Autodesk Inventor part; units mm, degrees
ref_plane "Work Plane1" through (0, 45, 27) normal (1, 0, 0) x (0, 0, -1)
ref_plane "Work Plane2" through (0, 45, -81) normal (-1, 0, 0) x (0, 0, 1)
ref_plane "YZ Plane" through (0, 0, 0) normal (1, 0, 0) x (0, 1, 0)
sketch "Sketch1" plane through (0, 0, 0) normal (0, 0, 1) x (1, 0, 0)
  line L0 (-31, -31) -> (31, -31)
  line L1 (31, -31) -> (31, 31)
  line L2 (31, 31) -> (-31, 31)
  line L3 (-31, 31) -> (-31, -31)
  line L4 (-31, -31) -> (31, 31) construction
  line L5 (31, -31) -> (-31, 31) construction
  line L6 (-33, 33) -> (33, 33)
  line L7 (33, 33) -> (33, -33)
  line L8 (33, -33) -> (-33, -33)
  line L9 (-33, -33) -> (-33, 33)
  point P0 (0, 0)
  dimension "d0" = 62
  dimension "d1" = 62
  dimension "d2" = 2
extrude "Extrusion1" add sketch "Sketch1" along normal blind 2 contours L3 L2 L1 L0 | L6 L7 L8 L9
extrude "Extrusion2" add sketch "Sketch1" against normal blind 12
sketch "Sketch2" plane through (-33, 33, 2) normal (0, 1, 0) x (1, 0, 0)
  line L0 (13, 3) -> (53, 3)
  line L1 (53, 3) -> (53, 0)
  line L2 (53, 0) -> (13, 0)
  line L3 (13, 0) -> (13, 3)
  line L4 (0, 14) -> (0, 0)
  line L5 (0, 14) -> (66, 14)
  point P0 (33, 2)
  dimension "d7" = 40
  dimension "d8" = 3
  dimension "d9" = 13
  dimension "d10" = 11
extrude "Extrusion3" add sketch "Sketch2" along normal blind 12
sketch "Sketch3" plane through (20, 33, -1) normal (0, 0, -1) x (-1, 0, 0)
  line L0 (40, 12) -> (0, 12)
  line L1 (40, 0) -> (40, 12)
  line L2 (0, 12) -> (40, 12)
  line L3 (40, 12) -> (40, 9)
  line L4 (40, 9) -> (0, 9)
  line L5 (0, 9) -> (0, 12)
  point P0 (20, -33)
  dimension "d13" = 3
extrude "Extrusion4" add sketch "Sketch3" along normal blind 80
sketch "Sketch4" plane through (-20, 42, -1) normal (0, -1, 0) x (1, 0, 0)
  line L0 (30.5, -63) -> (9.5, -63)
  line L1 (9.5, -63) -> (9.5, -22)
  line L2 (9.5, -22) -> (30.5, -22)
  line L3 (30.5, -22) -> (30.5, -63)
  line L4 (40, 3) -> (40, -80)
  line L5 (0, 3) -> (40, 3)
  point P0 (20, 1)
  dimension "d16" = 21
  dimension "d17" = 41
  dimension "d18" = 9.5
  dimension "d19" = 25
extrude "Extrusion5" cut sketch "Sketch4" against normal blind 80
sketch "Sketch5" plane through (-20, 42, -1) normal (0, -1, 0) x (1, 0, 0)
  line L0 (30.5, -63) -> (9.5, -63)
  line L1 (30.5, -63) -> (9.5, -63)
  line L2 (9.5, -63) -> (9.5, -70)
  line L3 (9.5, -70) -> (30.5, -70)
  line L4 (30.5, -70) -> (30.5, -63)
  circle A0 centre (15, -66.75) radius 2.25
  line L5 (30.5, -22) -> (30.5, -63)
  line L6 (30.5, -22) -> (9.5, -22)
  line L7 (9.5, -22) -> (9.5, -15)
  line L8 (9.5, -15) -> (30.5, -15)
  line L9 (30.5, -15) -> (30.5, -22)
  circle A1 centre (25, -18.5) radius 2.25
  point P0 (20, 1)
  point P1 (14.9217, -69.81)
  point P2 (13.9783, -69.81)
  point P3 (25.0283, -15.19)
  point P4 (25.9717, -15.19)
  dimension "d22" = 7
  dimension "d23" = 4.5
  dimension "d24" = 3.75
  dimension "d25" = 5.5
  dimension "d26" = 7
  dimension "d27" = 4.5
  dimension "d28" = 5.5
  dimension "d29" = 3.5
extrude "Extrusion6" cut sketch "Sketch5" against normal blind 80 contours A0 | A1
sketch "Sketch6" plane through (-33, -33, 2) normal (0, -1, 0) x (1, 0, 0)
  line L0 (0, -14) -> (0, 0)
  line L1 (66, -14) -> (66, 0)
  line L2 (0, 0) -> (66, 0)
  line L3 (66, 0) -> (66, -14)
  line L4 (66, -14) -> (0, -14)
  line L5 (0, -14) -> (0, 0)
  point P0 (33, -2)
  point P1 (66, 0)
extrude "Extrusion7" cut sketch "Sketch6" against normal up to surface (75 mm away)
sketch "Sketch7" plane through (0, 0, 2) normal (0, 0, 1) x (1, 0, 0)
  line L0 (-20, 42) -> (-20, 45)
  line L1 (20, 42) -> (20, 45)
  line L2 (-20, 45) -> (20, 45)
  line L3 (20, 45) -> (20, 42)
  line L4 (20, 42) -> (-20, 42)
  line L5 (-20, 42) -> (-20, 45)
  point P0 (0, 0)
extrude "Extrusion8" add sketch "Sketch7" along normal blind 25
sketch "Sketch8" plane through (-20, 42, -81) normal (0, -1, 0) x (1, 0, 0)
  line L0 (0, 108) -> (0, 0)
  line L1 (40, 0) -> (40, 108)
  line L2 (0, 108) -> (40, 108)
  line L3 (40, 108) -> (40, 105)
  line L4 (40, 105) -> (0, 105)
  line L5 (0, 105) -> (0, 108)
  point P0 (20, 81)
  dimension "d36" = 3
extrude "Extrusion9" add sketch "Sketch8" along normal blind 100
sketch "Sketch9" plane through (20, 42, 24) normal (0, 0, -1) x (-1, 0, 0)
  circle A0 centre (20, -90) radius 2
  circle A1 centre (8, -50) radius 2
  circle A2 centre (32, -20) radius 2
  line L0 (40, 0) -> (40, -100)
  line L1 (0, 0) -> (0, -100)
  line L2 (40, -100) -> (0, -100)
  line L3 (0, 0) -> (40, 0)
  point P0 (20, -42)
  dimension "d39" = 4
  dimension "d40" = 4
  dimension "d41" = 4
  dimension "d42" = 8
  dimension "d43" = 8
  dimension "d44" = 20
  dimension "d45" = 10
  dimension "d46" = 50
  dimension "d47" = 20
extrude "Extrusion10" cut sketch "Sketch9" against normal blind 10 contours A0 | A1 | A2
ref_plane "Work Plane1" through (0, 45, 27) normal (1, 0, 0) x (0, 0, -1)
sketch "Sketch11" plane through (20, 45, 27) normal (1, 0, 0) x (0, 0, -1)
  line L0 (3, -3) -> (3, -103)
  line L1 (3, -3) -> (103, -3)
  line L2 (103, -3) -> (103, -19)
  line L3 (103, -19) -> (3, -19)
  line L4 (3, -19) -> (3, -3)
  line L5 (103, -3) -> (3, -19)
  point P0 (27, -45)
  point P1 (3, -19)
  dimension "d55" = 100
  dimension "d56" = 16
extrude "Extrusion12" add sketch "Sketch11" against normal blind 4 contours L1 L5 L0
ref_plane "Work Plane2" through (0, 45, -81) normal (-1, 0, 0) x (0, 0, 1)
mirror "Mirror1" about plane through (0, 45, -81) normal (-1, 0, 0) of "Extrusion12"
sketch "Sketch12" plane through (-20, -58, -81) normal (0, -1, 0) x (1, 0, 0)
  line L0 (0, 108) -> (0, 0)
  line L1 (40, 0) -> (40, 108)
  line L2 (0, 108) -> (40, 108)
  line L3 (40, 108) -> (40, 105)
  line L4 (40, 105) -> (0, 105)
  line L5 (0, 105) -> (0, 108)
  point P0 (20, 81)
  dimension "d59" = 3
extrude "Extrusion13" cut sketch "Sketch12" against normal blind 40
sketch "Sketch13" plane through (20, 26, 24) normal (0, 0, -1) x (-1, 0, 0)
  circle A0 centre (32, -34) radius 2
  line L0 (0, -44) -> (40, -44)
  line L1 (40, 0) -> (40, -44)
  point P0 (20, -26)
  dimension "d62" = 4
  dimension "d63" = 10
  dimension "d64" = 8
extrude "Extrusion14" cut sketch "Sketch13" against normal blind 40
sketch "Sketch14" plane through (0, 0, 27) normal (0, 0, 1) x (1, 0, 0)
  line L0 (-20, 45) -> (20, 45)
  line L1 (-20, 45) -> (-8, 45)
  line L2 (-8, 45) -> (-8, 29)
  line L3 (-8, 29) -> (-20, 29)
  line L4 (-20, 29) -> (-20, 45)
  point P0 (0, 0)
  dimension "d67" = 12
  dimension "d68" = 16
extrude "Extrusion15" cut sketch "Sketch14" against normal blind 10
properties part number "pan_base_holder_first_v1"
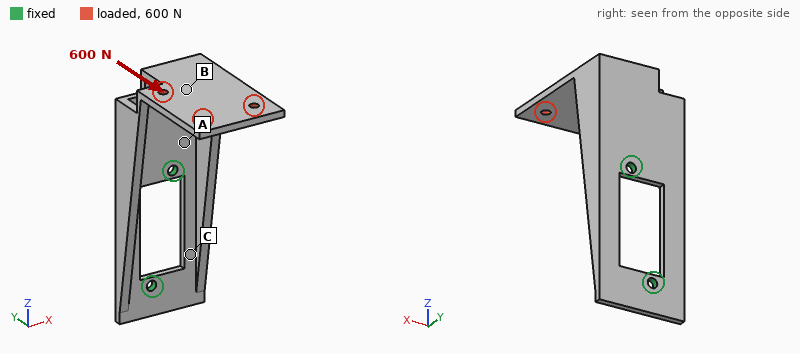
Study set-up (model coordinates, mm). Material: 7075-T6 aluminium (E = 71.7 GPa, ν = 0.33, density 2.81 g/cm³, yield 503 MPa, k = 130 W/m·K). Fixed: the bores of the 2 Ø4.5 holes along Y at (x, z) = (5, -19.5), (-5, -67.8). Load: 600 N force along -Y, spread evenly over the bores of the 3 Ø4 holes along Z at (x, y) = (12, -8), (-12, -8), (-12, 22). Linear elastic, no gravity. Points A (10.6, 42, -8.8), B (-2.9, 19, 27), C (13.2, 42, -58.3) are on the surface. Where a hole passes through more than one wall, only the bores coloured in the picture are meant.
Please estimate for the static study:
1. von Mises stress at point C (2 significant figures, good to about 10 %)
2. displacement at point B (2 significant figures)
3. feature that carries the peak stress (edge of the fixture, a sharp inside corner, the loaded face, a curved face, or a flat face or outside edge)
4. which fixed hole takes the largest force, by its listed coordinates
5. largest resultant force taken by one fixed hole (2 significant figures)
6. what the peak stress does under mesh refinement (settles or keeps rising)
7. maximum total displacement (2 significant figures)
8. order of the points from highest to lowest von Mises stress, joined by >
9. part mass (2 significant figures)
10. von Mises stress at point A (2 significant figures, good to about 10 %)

40 MPa
0.83 mm
edge of the fixture
(5, -19.5)
1.1 kN
keeps rising
1.5 mm
A > C > B
63 g
70 MPa
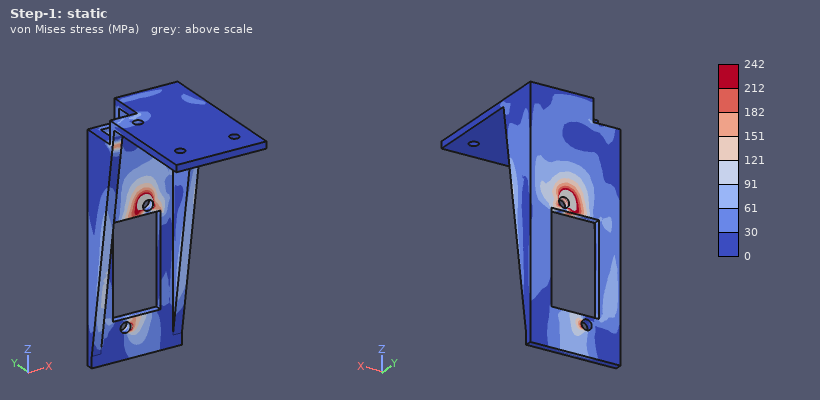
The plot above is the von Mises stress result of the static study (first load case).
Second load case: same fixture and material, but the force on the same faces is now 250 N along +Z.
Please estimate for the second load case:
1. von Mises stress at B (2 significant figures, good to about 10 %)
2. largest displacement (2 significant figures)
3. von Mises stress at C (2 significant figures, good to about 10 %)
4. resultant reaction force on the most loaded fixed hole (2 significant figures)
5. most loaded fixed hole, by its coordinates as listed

86 MPa
1.4 mm
20 MPa
390 N
(-5, -67.8)
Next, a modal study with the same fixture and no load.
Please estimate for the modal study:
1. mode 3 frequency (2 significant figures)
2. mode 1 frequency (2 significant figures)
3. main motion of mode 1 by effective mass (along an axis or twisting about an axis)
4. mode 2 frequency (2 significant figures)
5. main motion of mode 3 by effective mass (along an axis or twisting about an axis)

1200 Hz
570 Hz
along X
700 Hz
along Y
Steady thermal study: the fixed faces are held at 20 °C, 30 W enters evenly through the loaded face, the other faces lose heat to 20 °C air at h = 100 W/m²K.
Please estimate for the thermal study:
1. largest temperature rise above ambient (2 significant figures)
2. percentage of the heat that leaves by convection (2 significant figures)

56 K
83 %
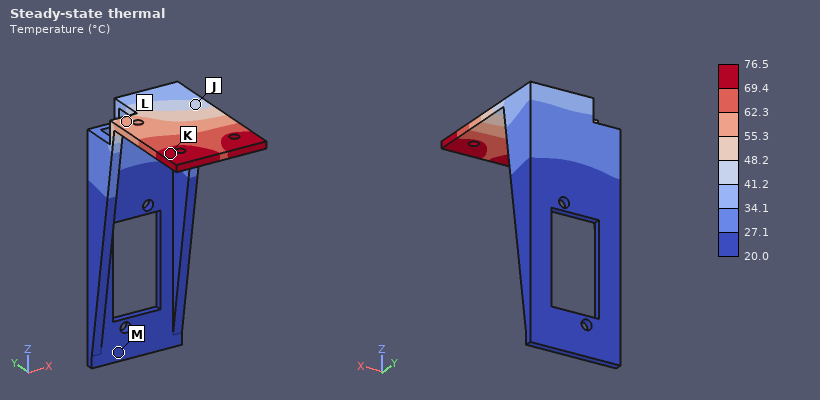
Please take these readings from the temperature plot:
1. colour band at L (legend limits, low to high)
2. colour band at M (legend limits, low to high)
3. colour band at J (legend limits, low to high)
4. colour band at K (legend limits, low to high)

55.3 to 62.3 °C
20.0 to 27.1 °C
41.2 to 48.2 °C
69.4 to 76.5 °C
